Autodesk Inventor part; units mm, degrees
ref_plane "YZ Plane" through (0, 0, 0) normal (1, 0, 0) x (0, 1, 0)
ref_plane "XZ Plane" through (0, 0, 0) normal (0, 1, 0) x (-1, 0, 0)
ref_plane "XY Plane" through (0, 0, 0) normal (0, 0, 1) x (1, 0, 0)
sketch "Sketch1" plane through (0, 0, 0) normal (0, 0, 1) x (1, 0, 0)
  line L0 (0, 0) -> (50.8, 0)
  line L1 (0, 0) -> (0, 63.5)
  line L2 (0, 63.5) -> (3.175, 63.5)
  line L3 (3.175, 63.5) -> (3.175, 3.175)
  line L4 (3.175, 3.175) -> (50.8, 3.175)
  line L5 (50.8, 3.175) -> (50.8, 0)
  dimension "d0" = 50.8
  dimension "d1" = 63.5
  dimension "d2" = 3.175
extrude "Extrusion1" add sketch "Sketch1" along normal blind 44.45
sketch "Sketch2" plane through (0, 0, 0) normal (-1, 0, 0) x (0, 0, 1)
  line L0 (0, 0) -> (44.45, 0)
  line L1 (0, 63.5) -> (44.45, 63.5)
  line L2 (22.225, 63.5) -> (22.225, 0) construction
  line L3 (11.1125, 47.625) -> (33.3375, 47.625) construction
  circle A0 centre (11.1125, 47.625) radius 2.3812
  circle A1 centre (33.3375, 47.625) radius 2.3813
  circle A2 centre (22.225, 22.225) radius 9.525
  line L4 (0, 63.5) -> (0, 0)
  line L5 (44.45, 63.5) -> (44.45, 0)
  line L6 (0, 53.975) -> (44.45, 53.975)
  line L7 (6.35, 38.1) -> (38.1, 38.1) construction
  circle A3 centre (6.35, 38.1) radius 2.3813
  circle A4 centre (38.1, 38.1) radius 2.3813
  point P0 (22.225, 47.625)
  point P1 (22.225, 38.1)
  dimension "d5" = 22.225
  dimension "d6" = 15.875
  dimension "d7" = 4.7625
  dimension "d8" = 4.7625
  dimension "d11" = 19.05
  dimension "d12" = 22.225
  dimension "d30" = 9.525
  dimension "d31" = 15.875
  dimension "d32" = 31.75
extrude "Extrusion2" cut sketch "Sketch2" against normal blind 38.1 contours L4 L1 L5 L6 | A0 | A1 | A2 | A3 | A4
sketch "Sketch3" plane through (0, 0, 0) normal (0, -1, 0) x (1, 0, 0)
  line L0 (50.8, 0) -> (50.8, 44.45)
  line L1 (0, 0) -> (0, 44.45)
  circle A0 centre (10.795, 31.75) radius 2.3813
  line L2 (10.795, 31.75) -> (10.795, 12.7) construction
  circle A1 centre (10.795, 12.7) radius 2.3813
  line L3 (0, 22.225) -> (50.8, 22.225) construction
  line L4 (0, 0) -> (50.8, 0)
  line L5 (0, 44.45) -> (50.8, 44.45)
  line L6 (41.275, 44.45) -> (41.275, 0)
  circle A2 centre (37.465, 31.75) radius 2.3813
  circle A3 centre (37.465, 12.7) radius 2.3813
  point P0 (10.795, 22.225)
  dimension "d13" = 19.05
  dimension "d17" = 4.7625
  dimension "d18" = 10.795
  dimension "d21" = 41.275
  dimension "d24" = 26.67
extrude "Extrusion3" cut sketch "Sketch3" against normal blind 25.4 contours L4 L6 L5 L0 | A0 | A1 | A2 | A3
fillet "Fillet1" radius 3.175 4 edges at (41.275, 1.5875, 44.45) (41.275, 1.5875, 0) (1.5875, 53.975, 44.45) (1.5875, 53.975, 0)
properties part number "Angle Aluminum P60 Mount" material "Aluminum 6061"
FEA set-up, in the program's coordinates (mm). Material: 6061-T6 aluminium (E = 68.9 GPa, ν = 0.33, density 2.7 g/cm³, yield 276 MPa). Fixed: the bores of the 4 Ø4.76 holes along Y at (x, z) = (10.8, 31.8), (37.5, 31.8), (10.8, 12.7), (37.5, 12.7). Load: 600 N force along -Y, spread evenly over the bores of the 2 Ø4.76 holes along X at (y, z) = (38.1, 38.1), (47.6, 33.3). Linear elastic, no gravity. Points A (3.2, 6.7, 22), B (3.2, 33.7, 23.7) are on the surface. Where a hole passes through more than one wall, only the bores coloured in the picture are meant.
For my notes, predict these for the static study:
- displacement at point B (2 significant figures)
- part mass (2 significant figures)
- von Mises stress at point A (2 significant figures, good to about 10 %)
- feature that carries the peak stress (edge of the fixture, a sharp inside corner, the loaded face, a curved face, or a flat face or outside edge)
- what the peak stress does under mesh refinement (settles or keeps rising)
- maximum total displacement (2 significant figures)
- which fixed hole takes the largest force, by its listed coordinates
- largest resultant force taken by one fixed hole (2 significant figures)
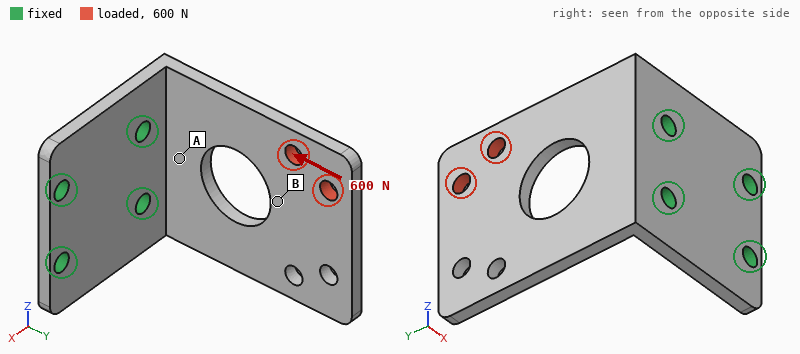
0.10 mm
31 g
20 MPa
edge of the fixture
keeps rising
0.19 mm
(10.8, 31.8)
660 N
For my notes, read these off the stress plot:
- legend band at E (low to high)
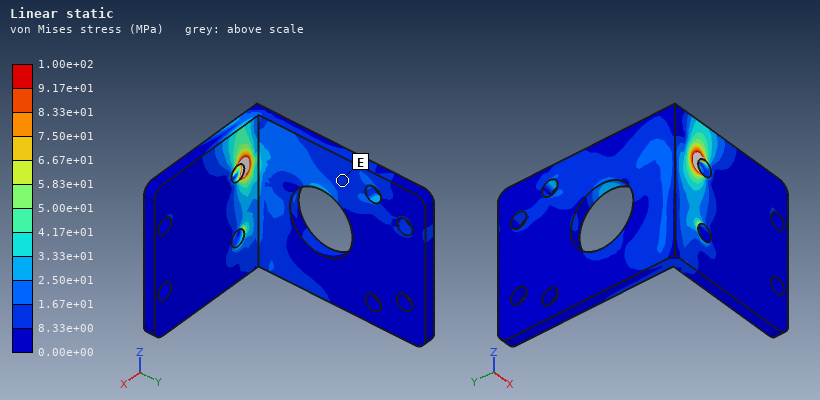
8.33e+00 to 1.67e+01 MPa
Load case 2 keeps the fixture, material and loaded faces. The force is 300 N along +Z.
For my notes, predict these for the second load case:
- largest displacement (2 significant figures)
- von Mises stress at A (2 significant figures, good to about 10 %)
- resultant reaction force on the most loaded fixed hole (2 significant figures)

0.14 mm
40 MPa
560 N
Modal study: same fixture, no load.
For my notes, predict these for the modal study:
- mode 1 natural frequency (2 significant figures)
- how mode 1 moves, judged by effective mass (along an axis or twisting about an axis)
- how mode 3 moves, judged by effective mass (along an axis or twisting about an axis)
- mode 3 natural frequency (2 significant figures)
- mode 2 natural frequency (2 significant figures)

740 Hz
along X
along Z
3000 Hz
2100 Hz
